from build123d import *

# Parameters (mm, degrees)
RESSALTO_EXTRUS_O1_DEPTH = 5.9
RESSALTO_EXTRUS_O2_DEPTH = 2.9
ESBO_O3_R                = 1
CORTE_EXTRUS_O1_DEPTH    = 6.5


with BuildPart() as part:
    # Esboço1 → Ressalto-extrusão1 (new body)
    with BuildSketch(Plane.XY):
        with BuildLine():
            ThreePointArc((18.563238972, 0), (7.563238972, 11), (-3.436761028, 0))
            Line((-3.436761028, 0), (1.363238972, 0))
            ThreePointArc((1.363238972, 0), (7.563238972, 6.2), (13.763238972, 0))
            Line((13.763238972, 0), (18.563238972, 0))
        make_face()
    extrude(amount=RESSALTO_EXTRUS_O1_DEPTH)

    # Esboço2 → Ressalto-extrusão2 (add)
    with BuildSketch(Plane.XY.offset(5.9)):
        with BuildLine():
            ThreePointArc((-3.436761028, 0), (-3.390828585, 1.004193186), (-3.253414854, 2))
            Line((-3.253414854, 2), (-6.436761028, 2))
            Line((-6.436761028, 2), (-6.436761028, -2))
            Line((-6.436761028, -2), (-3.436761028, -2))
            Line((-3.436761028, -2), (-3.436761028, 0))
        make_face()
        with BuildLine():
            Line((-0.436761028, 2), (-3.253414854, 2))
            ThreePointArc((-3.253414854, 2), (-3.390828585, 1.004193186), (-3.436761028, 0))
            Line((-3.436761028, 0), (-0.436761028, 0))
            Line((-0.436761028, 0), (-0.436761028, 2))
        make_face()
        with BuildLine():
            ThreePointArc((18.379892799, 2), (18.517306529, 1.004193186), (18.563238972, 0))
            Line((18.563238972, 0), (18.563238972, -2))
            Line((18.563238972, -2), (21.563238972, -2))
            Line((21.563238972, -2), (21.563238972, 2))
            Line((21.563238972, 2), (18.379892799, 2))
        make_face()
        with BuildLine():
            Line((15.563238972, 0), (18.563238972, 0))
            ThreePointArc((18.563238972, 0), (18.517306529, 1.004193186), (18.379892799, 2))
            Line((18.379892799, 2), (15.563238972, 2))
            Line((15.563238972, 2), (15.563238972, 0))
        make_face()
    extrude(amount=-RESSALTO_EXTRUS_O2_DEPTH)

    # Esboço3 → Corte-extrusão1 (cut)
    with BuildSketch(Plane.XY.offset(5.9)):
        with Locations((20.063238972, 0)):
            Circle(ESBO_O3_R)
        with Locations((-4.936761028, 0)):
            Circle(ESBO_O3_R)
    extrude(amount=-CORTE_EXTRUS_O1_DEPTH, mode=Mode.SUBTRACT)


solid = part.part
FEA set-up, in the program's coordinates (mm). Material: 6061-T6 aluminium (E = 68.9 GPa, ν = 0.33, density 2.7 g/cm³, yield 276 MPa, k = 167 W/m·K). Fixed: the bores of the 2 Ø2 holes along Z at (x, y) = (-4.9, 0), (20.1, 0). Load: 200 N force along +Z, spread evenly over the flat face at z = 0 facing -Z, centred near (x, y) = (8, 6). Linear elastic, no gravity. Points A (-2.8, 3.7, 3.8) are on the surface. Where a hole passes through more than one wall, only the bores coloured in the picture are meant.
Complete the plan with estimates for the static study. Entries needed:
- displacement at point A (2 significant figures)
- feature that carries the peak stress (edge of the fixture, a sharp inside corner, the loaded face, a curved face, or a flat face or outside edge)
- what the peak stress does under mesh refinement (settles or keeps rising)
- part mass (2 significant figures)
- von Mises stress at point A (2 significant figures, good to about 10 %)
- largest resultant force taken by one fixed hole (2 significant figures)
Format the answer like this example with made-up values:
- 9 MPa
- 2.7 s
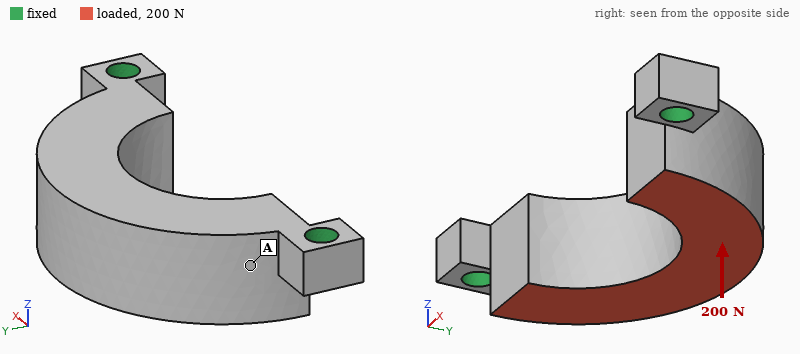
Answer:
- 16 µm
- a sharp inside corner
- keeps rising
- 2.2 g
- 35 MPa
- 100 N
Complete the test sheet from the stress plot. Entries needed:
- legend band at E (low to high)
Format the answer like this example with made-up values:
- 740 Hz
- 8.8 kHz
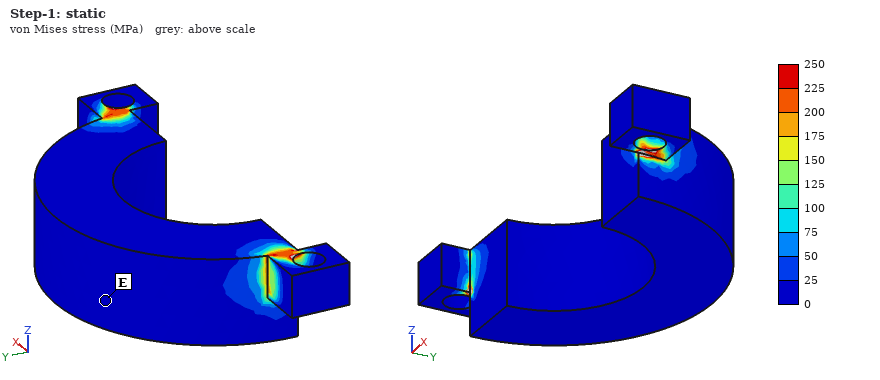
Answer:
- 0 to 25 MPa
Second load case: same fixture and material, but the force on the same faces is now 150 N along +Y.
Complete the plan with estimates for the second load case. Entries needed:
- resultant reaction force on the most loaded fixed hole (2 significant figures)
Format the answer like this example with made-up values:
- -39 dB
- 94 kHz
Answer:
- 90 N
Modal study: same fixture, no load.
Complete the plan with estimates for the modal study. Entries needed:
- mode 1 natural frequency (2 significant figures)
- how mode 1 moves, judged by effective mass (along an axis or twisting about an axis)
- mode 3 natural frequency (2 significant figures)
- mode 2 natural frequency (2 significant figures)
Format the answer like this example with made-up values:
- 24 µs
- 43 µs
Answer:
- 7600 Hz
- along Z
- 35 kHz
- 34 kHz
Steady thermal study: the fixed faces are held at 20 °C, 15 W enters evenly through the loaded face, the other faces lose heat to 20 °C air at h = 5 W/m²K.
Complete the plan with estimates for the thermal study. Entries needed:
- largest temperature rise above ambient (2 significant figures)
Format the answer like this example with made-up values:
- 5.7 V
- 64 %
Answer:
- 27 K
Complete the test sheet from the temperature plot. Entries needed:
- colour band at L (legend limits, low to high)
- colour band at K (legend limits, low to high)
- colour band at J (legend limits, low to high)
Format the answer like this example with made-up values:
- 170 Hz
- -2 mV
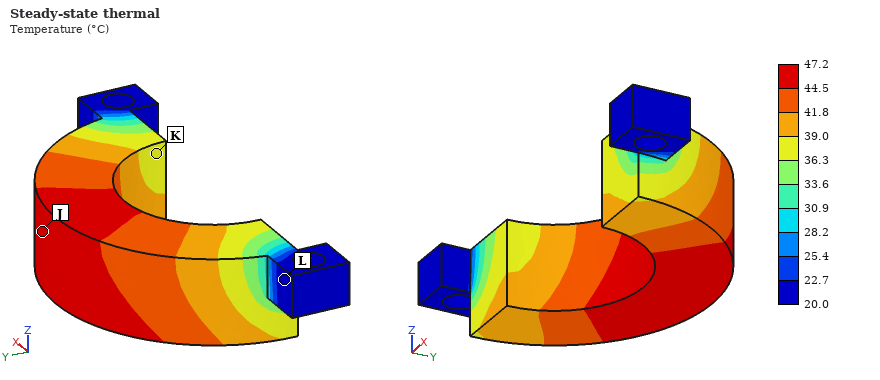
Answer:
- 20.0 to 22.7 °C
- 36.3 to 39.0 °C
- 44.5 to 47.2 °C
